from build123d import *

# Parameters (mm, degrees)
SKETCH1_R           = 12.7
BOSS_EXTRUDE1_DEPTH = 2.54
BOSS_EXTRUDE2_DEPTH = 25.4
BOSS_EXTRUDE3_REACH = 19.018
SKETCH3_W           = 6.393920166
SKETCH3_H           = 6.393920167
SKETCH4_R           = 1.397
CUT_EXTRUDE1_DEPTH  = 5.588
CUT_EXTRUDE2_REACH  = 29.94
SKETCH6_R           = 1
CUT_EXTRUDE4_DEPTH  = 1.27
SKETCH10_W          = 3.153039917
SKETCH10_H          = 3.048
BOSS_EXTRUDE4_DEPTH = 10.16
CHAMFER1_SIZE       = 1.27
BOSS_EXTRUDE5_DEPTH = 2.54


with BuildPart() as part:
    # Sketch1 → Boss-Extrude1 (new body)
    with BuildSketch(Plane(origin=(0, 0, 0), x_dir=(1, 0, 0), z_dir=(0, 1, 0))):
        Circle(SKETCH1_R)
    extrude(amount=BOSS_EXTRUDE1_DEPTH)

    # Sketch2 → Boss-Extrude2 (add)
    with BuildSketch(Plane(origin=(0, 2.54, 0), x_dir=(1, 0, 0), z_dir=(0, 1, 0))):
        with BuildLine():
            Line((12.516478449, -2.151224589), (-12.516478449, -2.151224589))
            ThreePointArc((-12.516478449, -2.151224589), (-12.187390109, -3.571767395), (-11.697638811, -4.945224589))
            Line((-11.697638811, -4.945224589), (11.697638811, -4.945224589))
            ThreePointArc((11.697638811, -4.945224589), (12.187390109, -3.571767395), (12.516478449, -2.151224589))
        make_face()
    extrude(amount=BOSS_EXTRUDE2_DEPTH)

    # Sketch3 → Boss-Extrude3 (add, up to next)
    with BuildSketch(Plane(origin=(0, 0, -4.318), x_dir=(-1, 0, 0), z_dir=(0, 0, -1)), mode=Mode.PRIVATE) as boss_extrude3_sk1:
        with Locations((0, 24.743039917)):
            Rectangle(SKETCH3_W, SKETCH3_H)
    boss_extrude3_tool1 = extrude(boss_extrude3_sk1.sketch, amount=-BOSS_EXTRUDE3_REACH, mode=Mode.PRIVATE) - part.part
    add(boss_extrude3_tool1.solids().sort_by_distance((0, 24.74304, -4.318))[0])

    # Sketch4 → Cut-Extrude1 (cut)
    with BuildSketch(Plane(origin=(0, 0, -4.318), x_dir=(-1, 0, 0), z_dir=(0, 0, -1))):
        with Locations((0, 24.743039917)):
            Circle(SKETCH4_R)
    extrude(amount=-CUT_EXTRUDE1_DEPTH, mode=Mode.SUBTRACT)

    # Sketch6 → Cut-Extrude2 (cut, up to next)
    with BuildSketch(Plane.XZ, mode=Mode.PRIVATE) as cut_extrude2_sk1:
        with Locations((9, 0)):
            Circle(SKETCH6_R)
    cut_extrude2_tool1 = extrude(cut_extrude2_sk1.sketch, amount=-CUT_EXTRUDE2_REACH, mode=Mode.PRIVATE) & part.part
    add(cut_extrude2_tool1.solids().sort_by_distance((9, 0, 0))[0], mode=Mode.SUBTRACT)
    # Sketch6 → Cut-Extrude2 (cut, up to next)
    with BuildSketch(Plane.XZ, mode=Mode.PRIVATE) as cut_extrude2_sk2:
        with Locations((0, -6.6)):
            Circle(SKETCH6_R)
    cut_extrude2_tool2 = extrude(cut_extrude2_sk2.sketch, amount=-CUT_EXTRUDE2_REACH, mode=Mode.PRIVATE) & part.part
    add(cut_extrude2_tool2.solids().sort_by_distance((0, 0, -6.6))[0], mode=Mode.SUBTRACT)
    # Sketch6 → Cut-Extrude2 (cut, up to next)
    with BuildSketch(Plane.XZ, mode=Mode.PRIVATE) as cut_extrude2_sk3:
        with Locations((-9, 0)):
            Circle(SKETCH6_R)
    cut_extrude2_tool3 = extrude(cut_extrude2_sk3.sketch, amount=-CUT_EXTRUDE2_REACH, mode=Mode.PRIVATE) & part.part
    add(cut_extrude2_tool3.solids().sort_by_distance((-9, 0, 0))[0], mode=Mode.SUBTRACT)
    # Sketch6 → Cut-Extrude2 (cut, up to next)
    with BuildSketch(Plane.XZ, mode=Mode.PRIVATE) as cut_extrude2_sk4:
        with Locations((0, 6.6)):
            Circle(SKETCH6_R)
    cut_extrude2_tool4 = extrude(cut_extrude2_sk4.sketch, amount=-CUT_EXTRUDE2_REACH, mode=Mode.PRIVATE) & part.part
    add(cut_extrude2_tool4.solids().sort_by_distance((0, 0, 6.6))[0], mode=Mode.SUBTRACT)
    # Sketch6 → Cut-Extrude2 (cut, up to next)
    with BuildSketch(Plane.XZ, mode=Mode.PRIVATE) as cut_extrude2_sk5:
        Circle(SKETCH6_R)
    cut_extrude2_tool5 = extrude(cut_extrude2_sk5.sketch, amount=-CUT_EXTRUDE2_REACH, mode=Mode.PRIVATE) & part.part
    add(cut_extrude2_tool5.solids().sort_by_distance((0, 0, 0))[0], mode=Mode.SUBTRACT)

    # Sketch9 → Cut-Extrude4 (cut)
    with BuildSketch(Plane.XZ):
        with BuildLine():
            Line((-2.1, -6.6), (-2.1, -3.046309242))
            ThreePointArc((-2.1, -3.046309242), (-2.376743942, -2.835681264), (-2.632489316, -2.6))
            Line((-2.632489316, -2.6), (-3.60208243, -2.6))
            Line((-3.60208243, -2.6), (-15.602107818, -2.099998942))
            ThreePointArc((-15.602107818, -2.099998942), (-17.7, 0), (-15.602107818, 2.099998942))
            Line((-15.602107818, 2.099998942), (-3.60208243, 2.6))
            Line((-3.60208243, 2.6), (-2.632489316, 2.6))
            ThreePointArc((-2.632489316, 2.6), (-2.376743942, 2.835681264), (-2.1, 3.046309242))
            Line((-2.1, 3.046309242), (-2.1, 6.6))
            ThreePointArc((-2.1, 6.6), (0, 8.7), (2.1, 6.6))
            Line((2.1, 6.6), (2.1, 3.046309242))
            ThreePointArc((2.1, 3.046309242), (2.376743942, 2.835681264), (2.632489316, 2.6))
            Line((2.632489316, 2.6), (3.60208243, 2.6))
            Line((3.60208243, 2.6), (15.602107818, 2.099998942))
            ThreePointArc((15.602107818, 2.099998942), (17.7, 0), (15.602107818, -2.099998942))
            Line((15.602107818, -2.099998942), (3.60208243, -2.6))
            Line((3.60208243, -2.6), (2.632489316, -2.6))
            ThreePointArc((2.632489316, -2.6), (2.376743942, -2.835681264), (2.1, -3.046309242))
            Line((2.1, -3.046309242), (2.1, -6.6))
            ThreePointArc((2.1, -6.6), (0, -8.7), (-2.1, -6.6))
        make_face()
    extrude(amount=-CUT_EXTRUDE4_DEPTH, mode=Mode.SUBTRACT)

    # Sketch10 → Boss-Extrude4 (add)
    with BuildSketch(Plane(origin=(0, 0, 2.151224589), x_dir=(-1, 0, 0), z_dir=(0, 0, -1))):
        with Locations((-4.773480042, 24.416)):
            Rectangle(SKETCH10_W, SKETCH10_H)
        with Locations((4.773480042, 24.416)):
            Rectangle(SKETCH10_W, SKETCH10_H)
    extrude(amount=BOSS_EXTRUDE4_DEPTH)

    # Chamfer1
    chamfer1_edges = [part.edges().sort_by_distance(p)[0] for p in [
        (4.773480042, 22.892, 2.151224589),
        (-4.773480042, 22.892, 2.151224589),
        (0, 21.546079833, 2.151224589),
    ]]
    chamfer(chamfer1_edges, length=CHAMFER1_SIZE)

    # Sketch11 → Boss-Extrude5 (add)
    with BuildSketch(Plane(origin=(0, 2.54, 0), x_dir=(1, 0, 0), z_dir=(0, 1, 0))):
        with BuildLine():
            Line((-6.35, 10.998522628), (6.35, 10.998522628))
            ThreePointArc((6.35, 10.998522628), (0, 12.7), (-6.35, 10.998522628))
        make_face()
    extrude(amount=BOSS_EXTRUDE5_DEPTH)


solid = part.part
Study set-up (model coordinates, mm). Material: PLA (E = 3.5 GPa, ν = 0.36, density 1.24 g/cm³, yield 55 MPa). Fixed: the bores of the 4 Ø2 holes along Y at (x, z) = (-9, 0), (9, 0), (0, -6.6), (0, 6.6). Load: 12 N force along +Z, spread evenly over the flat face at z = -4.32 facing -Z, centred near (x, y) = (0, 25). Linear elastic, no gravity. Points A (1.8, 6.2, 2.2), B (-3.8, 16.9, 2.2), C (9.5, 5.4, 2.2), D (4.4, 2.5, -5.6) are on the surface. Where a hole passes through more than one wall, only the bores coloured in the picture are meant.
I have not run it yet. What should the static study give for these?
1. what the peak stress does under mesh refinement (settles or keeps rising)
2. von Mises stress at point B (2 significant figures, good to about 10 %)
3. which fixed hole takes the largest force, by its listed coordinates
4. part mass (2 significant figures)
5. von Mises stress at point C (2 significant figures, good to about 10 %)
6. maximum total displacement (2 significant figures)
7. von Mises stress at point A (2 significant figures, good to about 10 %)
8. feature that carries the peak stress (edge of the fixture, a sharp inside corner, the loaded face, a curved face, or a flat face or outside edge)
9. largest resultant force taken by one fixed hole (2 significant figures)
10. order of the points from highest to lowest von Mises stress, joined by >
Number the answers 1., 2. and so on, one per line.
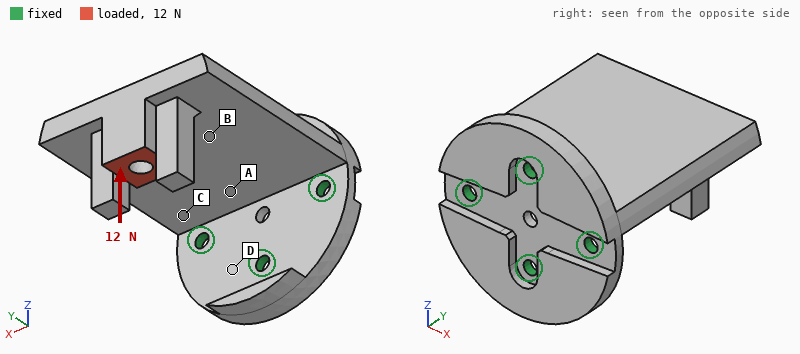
1. keeps rising
2. 2.7 MPa
3. (0, 6.6)
4. 4.0 g
5. 7.5 MPa
6. 0.50 mm
7. 5.6 MPa
8. edge of the fixture
9. 45 N
10. C > A > B > D
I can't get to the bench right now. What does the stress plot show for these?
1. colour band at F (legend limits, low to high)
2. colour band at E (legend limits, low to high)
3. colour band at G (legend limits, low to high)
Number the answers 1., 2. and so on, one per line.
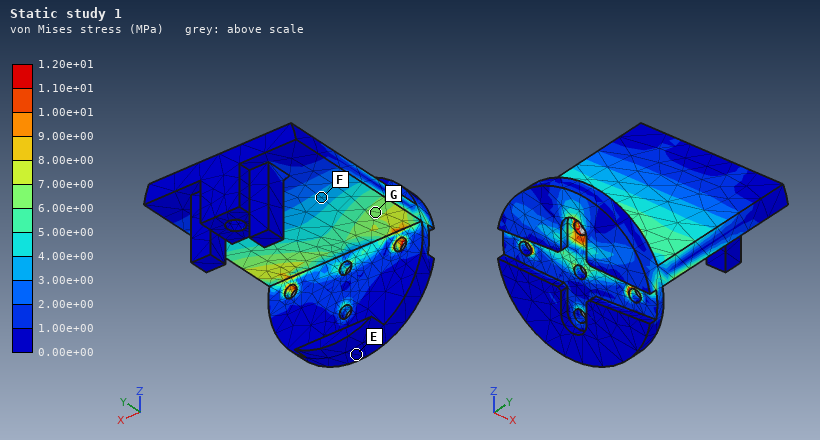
1. 3.00e+00 to 4.00e+00 MPa
2. 0.00e+00 to 1.00e+00 MPa
3. 6.00e+00 to 7.00e+00 MPa
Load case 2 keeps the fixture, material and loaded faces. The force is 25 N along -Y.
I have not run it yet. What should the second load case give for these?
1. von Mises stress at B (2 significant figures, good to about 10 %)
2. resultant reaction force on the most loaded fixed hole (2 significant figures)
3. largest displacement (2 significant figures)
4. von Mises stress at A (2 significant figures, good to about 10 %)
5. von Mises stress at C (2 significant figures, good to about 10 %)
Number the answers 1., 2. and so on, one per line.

1. 6.3 MPa
2. 22 N
3. 0.54 mm
4. 5.2 MPa
5. 6.9 MPa
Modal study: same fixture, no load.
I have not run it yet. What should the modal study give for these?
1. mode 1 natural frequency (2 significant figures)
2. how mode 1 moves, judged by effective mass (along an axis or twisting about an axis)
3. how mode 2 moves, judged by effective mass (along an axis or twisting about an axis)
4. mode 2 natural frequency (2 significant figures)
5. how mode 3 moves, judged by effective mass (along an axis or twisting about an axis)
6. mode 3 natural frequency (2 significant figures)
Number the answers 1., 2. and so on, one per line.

1. 740 Hz
2. along Z
3. along X
4. 1800 Hz
5. along X
6. 3100 Hz
